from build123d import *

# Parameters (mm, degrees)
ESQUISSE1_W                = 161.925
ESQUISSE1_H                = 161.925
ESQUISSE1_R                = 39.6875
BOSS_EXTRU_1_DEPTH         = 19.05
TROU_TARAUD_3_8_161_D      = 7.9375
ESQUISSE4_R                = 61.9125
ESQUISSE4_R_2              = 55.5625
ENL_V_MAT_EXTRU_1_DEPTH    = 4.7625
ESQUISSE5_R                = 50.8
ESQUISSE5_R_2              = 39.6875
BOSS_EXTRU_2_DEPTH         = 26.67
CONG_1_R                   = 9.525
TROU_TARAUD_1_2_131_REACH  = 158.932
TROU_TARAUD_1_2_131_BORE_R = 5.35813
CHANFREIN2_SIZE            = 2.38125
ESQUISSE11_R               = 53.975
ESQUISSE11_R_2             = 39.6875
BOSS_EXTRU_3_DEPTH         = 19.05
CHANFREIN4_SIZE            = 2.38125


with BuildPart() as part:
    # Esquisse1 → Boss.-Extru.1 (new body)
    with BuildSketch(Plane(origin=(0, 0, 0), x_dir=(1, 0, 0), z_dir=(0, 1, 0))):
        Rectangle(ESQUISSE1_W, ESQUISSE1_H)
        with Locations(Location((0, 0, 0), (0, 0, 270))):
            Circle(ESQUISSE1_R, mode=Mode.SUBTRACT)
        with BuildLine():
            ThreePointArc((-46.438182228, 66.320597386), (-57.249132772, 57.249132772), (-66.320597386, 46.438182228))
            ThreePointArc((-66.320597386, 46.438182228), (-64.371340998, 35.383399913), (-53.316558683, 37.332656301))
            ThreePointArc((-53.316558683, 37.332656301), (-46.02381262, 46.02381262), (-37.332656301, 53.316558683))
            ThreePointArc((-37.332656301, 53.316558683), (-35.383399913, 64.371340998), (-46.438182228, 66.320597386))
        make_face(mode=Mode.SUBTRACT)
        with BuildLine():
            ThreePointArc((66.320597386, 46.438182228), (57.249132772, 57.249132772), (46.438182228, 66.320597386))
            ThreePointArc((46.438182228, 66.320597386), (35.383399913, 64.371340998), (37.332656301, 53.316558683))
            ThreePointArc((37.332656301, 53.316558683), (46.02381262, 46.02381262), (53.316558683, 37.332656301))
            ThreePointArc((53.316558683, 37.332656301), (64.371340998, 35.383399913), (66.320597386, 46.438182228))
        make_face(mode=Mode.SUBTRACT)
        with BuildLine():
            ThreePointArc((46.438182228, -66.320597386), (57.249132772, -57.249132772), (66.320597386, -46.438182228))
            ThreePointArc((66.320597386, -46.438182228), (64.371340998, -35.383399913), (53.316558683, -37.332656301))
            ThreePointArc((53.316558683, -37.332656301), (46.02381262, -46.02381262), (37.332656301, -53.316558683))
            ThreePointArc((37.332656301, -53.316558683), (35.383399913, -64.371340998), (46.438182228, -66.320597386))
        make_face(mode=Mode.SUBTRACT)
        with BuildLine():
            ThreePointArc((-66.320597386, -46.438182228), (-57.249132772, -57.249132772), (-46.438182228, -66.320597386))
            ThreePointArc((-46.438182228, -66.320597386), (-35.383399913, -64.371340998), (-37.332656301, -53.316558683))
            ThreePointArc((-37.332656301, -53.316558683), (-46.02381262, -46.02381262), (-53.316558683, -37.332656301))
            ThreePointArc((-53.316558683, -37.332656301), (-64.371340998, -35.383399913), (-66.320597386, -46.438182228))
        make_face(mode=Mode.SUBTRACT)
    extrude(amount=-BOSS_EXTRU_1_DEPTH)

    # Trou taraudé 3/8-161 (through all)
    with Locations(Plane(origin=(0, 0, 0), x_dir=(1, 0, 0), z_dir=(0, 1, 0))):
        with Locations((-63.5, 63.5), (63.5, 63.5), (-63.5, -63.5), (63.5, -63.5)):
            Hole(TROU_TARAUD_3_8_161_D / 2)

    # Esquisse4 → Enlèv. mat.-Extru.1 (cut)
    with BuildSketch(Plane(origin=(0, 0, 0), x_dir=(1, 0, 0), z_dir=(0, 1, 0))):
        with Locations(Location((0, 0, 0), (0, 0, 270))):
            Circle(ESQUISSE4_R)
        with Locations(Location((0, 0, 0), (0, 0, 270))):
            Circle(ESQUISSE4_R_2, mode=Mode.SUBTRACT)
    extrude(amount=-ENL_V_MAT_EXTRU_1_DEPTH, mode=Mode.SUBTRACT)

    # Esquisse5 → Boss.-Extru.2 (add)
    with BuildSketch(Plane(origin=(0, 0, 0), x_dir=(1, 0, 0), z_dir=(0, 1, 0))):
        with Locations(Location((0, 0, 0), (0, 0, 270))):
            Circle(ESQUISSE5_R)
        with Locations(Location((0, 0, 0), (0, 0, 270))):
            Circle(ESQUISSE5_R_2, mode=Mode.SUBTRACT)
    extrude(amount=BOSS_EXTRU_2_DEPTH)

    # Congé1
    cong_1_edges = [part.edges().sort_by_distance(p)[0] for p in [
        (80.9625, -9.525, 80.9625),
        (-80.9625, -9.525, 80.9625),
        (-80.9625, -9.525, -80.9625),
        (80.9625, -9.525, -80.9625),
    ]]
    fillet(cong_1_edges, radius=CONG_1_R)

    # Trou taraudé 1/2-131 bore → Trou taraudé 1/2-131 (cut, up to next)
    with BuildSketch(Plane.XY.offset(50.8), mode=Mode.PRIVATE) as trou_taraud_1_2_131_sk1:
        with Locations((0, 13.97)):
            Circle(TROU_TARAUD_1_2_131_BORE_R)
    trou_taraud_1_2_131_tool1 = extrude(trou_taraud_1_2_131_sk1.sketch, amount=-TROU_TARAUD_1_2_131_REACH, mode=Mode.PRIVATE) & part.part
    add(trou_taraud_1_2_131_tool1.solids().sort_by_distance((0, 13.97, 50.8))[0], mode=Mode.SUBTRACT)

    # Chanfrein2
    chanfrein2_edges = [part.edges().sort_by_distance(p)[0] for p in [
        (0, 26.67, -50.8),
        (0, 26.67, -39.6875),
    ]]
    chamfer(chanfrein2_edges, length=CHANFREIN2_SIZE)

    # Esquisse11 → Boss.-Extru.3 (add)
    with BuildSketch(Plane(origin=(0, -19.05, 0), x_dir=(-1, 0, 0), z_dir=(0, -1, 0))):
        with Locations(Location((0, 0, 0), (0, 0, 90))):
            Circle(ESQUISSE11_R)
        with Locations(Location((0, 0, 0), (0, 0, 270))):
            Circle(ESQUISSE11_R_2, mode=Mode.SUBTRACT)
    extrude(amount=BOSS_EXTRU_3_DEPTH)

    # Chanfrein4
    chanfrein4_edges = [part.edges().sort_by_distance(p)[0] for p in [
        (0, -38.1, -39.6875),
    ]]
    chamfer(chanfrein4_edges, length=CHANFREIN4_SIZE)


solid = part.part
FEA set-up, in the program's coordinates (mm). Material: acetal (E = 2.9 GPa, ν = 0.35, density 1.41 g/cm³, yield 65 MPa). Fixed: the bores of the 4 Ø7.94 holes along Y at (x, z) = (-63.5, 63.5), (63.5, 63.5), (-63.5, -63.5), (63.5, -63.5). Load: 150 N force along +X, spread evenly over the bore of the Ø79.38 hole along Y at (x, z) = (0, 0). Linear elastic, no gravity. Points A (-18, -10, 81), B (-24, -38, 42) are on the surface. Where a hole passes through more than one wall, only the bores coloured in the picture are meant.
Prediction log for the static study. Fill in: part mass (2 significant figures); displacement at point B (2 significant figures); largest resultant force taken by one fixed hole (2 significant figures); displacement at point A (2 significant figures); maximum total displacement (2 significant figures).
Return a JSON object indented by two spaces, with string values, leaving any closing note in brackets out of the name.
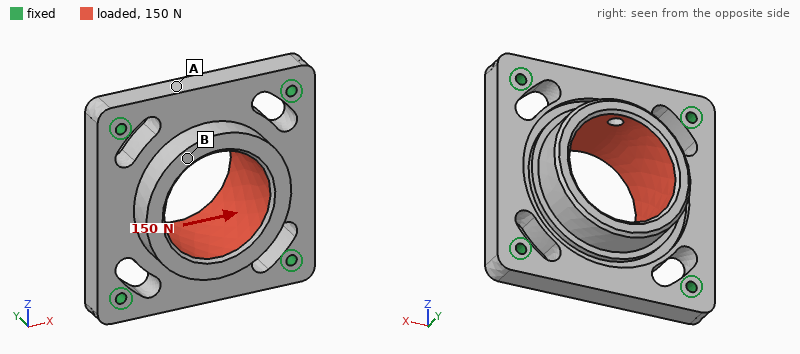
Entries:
{
  "part mass": "710 g",
  "displacement at point B": "2.9 µm",
  "largest resultant force taken by one fixed hole": "38 N",
  "displacement at point A": "1.4 µm",
  "maximum total displacement": "5.0 µm"
}
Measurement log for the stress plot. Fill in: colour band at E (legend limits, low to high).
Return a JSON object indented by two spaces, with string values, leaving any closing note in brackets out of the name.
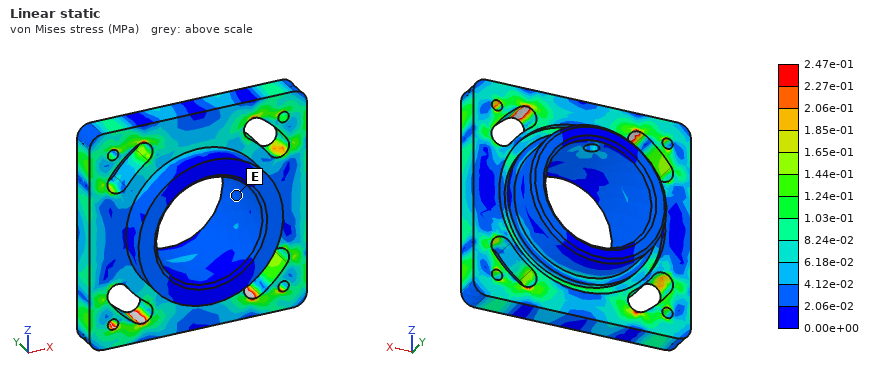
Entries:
{
  "colour band at E": "2.06e-02 to 4.12e-02 MPa"
}
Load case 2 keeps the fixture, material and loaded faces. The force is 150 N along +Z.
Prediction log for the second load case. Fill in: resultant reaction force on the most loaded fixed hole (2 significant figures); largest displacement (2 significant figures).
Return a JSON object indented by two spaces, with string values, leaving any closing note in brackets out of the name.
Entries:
{
  "resultant reaction force on the most loaded fixed hole": "38 N",
  "largest displacement": "5.0 µm"
}
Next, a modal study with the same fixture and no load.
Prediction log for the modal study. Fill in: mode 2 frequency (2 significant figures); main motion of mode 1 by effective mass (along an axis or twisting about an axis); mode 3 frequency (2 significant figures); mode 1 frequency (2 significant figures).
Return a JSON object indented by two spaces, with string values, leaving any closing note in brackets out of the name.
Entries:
{
  "mode 2 frequency": "1100 Hz",
  "main motion of mode 1 by effective mass": "along Y",
  "mode 3 frequency": "1100 Hz",
  "mode 1 frequency": "740 Hz"
}
